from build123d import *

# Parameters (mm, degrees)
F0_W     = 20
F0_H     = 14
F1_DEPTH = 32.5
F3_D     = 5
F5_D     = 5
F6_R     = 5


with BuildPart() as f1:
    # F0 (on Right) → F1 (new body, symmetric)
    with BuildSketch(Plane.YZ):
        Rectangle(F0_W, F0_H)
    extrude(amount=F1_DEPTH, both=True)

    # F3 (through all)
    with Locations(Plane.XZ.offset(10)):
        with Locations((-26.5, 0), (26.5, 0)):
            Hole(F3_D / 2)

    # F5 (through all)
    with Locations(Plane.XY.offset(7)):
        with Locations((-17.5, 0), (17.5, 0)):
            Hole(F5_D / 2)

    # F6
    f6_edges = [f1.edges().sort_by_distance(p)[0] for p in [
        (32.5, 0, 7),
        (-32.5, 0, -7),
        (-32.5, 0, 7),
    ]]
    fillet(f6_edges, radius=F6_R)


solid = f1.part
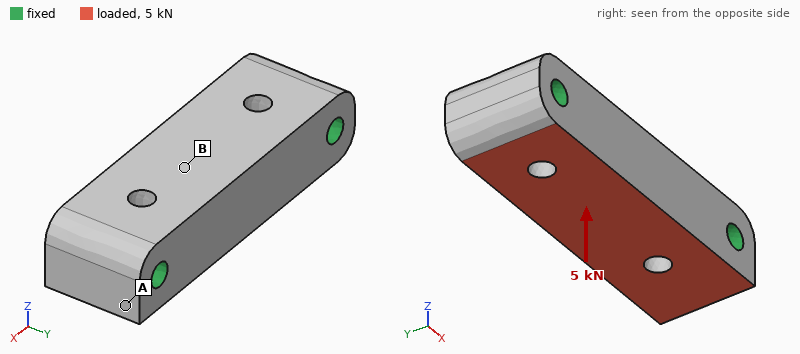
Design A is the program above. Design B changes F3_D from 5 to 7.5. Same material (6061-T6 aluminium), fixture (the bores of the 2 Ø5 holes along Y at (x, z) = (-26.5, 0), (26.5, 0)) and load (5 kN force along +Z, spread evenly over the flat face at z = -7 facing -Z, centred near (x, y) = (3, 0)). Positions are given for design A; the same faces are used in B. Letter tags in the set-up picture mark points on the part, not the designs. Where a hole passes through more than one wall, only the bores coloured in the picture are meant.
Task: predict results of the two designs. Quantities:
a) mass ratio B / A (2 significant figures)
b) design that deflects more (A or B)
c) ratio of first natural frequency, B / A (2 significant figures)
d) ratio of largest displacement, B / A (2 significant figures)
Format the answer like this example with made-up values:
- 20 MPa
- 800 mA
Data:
- 0.94
- A
- 1.2
- 0.76
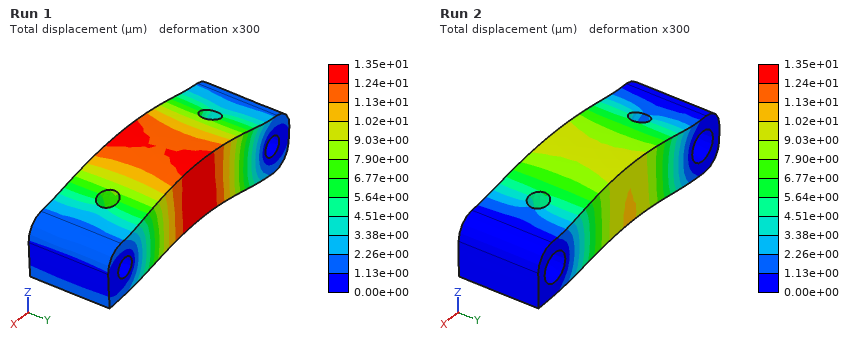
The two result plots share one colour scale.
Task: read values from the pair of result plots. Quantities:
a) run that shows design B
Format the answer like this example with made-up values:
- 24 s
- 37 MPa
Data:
- Run 2
